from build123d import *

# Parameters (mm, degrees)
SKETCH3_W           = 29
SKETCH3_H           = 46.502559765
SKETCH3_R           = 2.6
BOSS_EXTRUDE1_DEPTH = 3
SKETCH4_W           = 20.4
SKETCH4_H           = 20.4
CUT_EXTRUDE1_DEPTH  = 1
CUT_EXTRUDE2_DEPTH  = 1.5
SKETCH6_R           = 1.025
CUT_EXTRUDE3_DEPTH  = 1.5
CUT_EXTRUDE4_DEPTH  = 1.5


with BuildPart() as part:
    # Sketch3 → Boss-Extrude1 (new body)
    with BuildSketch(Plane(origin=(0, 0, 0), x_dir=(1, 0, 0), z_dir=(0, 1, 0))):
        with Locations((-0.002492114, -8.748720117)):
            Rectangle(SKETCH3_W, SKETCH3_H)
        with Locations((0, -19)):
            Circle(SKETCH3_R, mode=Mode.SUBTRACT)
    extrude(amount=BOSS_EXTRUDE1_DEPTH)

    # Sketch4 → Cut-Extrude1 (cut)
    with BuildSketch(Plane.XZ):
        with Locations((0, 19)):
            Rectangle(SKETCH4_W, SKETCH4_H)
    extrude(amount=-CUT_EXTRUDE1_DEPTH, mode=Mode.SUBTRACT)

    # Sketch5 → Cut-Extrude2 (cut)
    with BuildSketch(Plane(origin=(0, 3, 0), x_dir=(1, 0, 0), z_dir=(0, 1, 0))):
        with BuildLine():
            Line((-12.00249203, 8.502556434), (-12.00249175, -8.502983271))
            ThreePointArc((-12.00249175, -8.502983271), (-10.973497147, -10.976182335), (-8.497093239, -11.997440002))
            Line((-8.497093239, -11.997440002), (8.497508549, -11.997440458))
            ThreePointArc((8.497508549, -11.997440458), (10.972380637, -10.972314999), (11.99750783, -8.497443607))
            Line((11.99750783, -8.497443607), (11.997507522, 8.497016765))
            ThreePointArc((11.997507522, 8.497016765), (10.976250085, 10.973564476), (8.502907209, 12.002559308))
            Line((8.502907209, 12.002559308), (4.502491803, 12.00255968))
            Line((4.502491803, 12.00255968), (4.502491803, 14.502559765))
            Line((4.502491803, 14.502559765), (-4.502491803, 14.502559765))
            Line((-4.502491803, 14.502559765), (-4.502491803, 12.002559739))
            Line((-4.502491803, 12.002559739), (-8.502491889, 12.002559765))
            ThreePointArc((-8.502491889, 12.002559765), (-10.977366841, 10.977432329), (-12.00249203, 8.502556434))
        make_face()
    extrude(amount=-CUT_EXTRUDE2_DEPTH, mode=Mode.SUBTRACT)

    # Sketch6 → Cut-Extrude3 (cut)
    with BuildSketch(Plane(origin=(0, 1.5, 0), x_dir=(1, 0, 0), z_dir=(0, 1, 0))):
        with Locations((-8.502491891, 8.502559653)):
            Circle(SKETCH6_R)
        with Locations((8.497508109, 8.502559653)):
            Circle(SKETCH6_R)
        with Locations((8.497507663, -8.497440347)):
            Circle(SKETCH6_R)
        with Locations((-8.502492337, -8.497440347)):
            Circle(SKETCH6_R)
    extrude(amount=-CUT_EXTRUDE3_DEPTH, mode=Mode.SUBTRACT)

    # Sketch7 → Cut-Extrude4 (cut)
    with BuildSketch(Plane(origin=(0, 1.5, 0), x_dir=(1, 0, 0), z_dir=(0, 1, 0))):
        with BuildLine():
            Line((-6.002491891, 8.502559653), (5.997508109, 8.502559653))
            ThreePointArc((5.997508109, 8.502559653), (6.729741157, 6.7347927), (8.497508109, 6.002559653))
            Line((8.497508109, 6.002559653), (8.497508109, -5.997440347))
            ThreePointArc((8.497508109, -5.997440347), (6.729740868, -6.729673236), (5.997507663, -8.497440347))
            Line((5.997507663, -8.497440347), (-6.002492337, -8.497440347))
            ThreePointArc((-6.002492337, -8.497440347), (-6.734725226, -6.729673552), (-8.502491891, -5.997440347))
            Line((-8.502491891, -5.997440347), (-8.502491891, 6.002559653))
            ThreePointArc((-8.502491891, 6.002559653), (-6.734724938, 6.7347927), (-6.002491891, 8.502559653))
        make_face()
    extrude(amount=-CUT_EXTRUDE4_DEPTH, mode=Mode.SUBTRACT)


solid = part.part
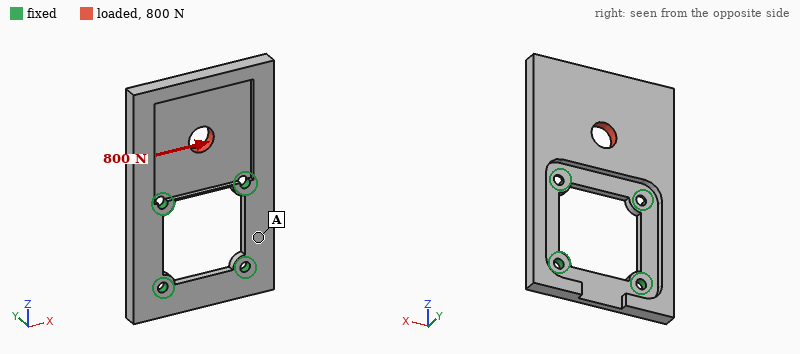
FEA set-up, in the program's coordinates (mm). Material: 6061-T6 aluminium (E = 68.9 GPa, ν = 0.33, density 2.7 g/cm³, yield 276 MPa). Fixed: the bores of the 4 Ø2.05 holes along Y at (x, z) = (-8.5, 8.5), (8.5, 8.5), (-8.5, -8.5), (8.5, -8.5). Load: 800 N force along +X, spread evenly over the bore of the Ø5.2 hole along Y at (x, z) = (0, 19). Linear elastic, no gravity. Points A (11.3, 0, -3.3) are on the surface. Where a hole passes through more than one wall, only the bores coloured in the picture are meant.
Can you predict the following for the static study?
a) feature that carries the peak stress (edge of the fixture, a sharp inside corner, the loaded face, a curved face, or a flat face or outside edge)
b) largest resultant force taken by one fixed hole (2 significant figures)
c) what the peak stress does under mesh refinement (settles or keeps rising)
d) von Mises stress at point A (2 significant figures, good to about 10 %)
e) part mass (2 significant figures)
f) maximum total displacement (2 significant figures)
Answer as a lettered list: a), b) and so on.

a) edge of the fixture
b) 500 N
c) keeps rising
d) 20 MPa
e) 6.2 g
f) 25 µm
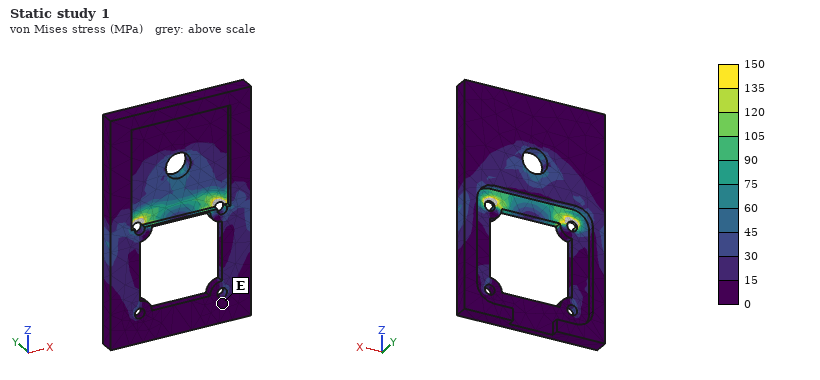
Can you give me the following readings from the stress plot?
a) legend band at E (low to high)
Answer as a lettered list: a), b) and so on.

a) 0 to 15 MPa
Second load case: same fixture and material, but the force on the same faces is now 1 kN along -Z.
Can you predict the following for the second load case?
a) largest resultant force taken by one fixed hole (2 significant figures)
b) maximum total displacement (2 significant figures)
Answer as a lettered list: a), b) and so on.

a) 430 N
b) 0.16 mm
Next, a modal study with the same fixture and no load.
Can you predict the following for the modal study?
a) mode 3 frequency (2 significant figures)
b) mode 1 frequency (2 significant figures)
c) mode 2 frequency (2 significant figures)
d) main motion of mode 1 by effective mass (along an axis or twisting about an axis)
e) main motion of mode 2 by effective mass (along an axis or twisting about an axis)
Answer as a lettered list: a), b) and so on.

a) 14 kHz
b) 1900 Hz
c) 4800 Hz
d) along Y
e) twisting about Z
